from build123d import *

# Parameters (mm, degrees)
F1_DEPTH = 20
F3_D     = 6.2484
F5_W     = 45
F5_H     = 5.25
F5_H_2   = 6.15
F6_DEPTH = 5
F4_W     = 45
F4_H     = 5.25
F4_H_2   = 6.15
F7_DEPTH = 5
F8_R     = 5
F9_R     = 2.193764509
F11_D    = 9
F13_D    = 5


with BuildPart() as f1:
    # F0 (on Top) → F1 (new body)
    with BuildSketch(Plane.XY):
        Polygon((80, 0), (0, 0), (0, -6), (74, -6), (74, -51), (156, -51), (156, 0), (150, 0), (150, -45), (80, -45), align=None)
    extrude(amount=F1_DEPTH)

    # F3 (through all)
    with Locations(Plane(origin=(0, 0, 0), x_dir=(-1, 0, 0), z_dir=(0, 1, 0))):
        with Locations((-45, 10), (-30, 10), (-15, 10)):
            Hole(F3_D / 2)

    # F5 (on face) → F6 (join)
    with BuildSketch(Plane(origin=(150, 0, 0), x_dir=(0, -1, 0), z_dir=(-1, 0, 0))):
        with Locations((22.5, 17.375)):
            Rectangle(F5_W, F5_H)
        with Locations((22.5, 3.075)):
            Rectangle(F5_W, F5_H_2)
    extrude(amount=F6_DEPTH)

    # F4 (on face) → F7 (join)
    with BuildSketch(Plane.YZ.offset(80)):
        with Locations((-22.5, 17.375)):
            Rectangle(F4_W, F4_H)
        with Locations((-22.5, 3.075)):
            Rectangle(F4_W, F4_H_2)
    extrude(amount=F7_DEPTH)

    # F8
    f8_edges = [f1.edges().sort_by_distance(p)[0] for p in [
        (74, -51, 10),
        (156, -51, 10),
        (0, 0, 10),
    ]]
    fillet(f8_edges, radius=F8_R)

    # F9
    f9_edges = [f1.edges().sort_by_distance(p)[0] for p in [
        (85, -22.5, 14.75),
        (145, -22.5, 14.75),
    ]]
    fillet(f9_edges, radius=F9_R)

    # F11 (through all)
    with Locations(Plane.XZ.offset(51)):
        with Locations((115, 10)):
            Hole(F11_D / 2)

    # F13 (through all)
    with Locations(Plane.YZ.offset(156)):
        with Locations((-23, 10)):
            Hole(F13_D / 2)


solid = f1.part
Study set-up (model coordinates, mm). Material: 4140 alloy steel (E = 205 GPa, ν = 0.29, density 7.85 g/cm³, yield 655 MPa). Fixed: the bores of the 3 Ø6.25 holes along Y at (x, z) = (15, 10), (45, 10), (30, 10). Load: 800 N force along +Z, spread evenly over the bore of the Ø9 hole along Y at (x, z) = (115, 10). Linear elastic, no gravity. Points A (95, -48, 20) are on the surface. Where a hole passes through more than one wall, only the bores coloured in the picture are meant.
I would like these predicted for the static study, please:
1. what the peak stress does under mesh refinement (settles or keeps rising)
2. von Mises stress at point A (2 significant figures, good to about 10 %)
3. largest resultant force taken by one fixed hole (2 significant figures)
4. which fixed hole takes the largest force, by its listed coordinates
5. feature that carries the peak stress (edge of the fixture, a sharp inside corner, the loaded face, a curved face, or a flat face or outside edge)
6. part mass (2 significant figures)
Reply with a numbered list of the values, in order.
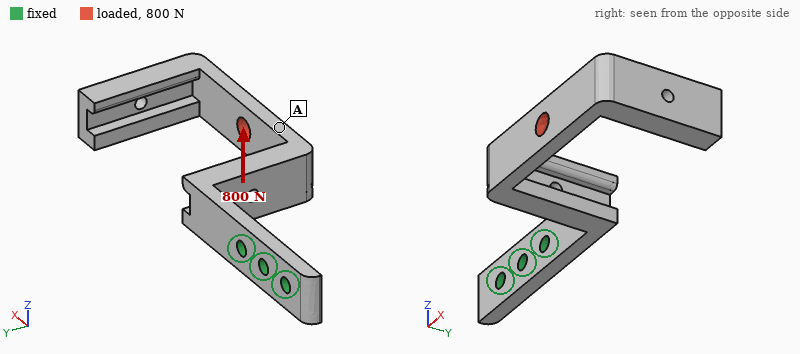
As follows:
1. keeps rising
2. 40 MPa
3. 2.4 kN
4. (45, 10)
5. edge of the fixture
6. 260 g
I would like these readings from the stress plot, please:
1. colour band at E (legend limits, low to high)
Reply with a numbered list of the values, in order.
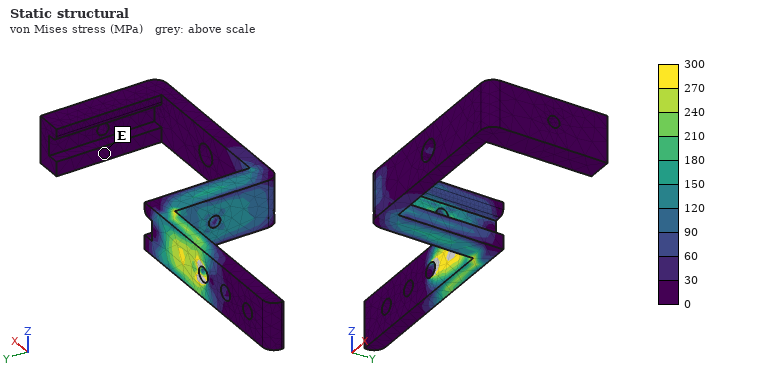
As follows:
1. 0 to 30 MPa
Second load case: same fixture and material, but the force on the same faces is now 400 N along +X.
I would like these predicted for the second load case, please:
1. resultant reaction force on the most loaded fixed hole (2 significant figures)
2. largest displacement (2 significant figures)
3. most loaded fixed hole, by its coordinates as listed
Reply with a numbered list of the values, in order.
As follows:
1. 400 N
2. 0.87 mm
3. (45, 10)
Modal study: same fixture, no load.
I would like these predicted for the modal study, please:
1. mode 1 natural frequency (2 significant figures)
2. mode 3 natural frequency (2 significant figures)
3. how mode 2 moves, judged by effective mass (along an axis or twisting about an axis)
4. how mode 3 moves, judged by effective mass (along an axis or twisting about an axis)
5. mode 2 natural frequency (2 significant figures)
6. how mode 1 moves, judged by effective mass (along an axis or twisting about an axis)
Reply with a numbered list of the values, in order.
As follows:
1. 210 Hz
2. 560 Hz
3. along Z
4. along X
5. 340 Hz
6. along Y
